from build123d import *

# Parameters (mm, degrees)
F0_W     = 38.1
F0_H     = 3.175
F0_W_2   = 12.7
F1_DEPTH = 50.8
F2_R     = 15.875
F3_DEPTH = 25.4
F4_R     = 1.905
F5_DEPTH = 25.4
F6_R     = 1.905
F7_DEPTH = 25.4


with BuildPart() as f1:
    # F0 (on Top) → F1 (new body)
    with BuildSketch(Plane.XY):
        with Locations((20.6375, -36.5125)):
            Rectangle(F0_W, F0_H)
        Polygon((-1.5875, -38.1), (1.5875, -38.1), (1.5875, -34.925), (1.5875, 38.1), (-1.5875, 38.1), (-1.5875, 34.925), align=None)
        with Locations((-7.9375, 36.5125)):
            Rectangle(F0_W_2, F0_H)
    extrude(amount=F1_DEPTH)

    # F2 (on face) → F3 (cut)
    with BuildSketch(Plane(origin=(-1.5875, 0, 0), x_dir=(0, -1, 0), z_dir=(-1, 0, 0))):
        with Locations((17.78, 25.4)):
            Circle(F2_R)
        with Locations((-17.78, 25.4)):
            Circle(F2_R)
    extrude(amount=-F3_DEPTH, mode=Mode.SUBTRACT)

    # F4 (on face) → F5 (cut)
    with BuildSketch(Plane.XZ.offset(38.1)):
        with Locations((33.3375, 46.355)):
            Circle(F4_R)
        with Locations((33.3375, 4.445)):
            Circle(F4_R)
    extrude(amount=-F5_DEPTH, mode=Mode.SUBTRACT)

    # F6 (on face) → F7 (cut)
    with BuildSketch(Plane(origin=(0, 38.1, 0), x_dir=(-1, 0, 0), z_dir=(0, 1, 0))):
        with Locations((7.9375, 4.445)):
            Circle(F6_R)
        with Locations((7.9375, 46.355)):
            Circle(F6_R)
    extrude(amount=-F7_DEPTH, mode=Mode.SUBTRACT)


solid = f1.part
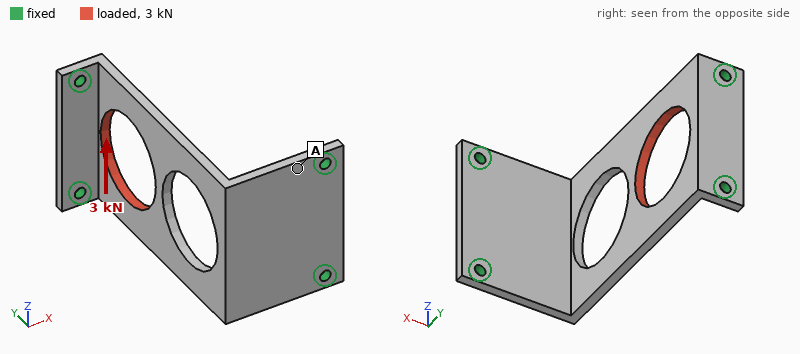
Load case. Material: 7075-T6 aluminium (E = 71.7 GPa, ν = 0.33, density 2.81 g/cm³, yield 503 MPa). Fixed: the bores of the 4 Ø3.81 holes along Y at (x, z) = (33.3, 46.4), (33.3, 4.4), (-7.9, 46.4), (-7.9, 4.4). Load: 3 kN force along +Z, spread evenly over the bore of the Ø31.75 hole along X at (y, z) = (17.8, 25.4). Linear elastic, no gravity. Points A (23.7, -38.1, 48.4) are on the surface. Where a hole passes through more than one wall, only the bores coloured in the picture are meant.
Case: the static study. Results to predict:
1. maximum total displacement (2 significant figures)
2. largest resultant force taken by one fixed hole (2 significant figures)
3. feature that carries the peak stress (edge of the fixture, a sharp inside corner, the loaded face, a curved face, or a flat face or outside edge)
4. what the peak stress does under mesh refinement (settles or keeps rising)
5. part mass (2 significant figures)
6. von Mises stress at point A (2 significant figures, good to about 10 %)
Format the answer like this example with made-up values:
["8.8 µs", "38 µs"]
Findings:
["79 µm", "1.2 kN", "edge of the fixture", "keeps rising", "43 g", "14 MPa"]
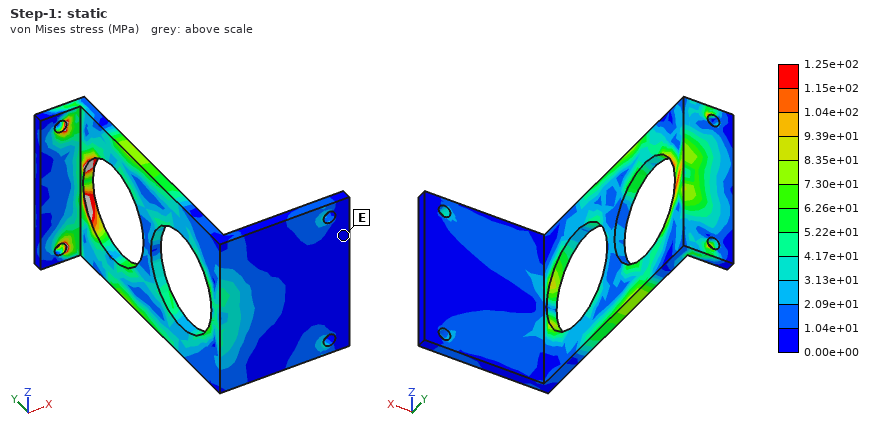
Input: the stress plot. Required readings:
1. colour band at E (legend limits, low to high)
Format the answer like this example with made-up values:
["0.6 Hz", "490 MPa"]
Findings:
["0.00e+00 to 1.04e+01 MPa"]
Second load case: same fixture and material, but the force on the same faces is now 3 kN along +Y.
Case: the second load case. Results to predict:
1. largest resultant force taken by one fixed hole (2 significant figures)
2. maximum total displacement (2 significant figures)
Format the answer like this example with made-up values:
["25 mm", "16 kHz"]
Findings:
["1.5 kN", "0.18 mm"]
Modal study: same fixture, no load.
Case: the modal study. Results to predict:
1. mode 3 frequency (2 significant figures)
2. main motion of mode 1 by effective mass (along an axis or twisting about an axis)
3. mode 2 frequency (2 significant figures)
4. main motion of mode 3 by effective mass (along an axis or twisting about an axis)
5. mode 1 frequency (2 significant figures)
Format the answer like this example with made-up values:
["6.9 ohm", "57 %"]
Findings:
["5700 Hz", "along X", "3200 Hz", "along Y", "2400 Hz"]
